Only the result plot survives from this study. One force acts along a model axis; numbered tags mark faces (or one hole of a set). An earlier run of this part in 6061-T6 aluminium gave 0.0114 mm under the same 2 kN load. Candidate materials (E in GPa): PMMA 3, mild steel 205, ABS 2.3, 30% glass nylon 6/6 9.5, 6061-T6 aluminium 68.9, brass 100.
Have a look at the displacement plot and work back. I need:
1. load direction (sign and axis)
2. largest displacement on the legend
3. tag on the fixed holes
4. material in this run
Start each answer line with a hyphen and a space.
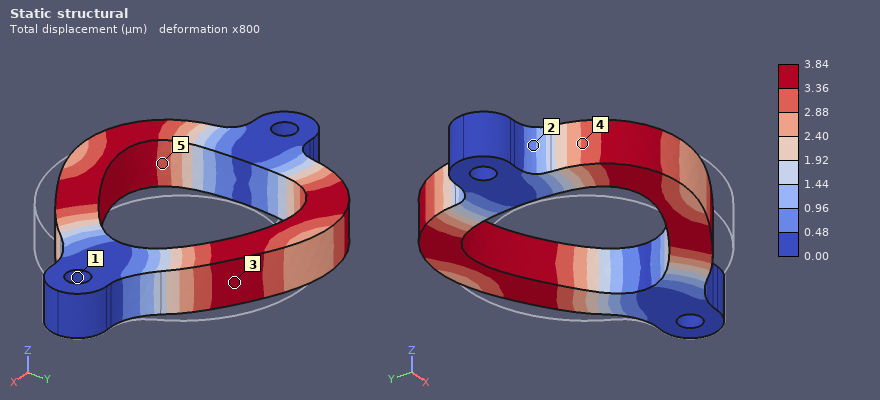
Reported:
- -X
- 3.84 µm
- 1
- mild steel
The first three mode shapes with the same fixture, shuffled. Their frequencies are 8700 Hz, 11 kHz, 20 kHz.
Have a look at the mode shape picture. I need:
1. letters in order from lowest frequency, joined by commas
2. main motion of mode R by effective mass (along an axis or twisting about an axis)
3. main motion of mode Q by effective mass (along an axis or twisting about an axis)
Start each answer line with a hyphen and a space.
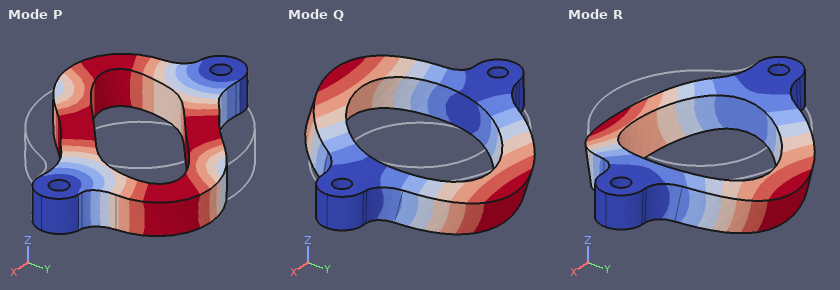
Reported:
- Q, R, P
- along Z
- twisting about X
